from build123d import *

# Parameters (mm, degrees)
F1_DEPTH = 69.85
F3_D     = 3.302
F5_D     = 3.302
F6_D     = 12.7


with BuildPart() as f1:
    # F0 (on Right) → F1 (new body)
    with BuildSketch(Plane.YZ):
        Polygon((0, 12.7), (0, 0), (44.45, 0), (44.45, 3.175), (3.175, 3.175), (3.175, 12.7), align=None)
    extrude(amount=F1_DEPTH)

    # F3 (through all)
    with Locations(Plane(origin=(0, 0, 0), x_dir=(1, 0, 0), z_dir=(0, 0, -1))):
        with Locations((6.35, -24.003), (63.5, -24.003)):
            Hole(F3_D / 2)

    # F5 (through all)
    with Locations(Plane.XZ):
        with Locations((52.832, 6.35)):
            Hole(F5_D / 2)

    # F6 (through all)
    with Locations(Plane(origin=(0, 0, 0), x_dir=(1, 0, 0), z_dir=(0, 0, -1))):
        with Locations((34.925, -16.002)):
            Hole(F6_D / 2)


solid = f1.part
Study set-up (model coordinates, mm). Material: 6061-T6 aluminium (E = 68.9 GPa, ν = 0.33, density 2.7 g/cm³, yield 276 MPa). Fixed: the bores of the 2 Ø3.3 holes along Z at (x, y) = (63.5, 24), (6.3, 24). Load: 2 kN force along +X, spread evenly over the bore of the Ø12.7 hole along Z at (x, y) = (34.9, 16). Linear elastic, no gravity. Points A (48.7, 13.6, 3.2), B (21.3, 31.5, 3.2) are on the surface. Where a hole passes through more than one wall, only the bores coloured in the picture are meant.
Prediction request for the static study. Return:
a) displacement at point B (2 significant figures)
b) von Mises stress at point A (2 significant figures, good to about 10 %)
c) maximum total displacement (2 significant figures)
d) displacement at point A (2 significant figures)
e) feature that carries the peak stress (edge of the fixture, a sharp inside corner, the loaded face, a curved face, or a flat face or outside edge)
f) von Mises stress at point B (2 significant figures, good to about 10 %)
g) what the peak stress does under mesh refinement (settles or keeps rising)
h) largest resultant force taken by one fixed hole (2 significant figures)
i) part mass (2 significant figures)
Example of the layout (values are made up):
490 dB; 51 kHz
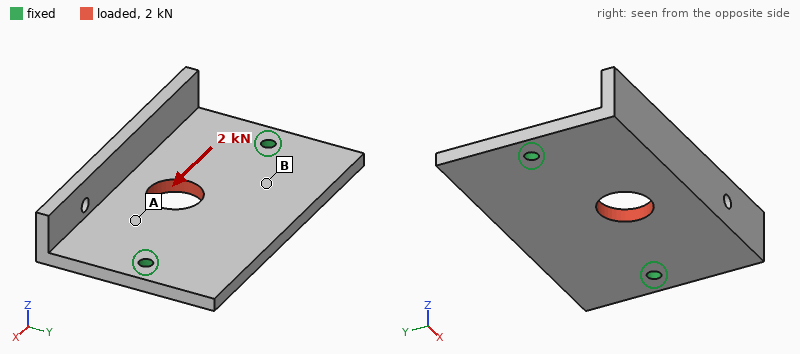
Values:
3.3 µm; 18 MPa; 10 µm; 6.8 µm; edge of the fixture; 6.9 MPa; keeps rising; 1.0 kN; 31 g
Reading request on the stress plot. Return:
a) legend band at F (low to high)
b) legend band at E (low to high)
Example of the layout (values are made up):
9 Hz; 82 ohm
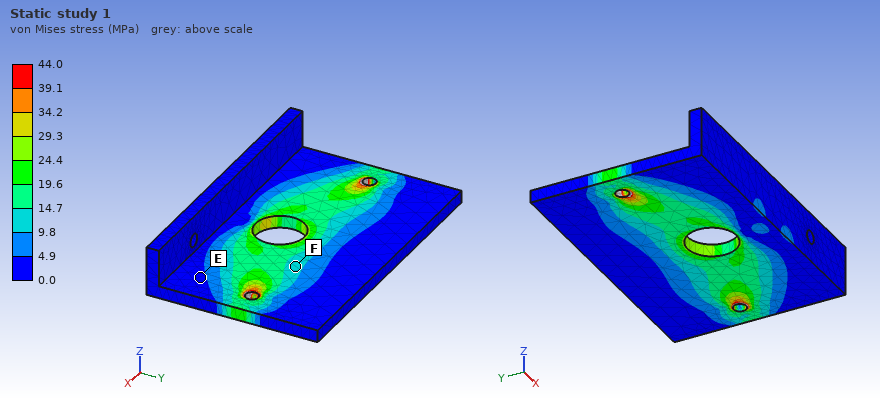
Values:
9.8 to 14.7 MPa; 0.0 to 4.9 MPa
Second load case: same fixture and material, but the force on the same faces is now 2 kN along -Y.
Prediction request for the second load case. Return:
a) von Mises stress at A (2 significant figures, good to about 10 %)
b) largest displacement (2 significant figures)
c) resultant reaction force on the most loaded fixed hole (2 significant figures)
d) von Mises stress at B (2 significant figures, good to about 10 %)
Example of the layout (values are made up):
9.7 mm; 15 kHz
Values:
19 MPa; 20 µm; 1.0 kN; 15 MPa
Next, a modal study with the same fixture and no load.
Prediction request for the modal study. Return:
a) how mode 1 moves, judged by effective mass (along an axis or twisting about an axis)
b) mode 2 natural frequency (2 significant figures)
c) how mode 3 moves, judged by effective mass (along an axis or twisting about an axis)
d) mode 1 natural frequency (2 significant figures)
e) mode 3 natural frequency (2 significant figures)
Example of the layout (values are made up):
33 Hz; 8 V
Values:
along Z; 3700 Hz; twisting about Y; 2100 Hz; 3900 Hz
